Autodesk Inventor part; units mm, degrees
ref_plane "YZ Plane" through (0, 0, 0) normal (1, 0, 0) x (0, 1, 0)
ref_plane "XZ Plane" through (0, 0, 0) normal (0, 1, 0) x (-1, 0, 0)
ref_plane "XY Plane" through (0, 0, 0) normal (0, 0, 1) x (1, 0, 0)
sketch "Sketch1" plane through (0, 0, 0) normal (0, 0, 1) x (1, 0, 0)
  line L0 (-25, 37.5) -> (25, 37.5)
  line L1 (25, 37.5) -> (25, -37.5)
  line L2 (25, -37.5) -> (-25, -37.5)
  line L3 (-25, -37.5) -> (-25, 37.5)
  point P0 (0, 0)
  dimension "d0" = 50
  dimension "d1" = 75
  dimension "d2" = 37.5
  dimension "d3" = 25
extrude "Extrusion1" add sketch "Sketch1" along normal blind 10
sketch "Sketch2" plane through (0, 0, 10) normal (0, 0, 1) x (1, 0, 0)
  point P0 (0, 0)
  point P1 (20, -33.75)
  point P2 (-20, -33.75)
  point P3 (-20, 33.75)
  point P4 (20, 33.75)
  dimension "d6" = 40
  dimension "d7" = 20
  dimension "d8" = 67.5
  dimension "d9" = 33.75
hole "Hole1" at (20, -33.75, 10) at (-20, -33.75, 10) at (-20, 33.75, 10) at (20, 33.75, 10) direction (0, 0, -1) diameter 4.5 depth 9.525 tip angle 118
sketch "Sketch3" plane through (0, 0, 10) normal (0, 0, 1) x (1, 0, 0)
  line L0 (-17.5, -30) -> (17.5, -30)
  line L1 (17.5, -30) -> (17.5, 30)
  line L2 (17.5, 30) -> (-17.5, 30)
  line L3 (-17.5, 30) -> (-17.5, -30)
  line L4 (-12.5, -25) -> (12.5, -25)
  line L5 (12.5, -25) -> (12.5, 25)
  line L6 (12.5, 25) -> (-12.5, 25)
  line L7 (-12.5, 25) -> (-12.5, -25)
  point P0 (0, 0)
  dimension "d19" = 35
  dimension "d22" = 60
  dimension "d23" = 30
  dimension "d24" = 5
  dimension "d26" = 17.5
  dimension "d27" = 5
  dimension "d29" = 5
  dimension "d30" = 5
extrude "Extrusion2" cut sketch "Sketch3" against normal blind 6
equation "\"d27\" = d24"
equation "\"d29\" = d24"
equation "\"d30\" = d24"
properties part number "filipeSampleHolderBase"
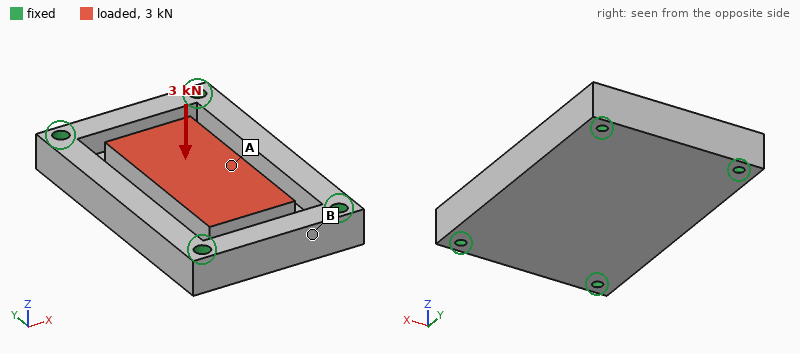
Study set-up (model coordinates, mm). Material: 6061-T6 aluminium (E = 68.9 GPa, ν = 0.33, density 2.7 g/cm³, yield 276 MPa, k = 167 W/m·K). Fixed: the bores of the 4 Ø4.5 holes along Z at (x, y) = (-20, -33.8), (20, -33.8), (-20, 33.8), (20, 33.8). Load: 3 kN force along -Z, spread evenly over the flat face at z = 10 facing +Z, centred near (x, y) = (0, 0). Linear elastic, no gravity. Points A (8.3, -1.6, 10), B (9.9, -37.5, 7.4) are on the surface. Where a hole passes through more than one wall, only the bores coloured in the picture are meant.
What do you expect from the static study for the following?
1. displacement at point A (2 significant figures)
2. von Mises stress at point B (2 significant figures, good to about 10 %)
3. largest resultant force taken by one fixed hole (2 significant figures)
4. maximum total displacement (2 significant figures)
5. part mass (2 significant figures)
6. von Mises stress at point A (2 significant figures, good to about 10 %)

29 µm
5.8 MPa
750 N
30 µm
86 g
19 MPa
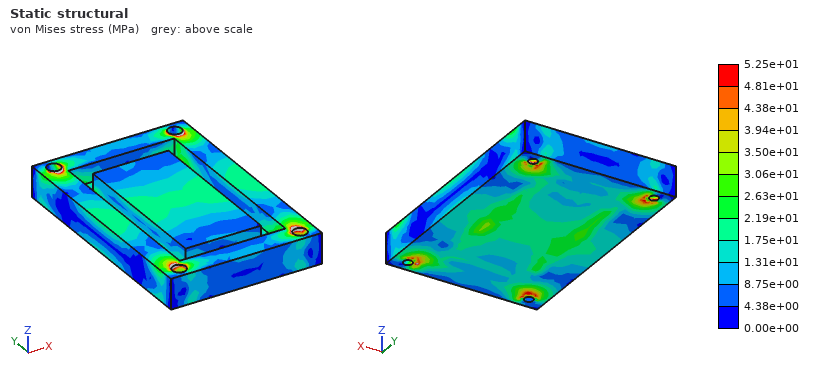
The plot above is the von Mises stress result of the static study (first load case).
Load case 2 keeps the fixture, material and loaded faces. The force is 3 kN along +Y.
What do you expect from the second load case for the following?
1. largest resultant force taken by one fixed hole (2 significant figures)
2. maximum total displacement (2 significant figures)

800 N
7.5 µm
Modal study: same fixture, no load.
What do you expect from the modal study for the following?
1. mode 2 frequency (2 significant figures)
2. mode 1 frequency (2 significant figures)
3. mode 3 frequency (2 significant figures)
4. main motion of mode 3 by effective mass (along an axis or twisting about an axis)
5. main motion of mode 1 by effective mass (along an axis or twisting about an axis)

11 kHz
7900 Hz
16 kHz
along X
along Z
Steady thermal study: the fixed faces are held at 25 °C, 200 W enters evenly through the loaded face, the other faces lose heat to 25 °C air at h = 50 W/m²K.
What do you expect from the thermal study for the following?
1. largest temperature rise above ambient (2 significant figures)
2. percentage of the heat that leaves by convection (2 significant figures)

54 K
6.4 %
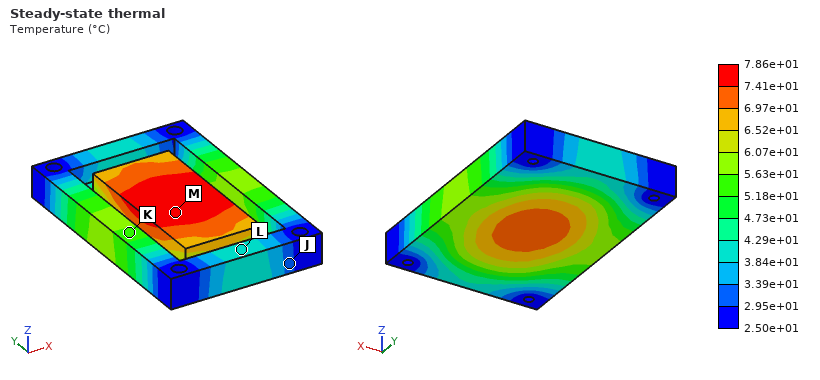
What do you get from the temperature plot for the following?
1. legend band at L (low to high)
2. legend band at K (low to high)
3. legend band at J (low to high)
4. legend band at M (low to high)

3.84e+01 to 4.29e+01 °C
5.18e+01 to 5.63e+01 °C
2.95e+01 to 3.39e+01 °C
7.41e+01 to 7.86e+01 °C
